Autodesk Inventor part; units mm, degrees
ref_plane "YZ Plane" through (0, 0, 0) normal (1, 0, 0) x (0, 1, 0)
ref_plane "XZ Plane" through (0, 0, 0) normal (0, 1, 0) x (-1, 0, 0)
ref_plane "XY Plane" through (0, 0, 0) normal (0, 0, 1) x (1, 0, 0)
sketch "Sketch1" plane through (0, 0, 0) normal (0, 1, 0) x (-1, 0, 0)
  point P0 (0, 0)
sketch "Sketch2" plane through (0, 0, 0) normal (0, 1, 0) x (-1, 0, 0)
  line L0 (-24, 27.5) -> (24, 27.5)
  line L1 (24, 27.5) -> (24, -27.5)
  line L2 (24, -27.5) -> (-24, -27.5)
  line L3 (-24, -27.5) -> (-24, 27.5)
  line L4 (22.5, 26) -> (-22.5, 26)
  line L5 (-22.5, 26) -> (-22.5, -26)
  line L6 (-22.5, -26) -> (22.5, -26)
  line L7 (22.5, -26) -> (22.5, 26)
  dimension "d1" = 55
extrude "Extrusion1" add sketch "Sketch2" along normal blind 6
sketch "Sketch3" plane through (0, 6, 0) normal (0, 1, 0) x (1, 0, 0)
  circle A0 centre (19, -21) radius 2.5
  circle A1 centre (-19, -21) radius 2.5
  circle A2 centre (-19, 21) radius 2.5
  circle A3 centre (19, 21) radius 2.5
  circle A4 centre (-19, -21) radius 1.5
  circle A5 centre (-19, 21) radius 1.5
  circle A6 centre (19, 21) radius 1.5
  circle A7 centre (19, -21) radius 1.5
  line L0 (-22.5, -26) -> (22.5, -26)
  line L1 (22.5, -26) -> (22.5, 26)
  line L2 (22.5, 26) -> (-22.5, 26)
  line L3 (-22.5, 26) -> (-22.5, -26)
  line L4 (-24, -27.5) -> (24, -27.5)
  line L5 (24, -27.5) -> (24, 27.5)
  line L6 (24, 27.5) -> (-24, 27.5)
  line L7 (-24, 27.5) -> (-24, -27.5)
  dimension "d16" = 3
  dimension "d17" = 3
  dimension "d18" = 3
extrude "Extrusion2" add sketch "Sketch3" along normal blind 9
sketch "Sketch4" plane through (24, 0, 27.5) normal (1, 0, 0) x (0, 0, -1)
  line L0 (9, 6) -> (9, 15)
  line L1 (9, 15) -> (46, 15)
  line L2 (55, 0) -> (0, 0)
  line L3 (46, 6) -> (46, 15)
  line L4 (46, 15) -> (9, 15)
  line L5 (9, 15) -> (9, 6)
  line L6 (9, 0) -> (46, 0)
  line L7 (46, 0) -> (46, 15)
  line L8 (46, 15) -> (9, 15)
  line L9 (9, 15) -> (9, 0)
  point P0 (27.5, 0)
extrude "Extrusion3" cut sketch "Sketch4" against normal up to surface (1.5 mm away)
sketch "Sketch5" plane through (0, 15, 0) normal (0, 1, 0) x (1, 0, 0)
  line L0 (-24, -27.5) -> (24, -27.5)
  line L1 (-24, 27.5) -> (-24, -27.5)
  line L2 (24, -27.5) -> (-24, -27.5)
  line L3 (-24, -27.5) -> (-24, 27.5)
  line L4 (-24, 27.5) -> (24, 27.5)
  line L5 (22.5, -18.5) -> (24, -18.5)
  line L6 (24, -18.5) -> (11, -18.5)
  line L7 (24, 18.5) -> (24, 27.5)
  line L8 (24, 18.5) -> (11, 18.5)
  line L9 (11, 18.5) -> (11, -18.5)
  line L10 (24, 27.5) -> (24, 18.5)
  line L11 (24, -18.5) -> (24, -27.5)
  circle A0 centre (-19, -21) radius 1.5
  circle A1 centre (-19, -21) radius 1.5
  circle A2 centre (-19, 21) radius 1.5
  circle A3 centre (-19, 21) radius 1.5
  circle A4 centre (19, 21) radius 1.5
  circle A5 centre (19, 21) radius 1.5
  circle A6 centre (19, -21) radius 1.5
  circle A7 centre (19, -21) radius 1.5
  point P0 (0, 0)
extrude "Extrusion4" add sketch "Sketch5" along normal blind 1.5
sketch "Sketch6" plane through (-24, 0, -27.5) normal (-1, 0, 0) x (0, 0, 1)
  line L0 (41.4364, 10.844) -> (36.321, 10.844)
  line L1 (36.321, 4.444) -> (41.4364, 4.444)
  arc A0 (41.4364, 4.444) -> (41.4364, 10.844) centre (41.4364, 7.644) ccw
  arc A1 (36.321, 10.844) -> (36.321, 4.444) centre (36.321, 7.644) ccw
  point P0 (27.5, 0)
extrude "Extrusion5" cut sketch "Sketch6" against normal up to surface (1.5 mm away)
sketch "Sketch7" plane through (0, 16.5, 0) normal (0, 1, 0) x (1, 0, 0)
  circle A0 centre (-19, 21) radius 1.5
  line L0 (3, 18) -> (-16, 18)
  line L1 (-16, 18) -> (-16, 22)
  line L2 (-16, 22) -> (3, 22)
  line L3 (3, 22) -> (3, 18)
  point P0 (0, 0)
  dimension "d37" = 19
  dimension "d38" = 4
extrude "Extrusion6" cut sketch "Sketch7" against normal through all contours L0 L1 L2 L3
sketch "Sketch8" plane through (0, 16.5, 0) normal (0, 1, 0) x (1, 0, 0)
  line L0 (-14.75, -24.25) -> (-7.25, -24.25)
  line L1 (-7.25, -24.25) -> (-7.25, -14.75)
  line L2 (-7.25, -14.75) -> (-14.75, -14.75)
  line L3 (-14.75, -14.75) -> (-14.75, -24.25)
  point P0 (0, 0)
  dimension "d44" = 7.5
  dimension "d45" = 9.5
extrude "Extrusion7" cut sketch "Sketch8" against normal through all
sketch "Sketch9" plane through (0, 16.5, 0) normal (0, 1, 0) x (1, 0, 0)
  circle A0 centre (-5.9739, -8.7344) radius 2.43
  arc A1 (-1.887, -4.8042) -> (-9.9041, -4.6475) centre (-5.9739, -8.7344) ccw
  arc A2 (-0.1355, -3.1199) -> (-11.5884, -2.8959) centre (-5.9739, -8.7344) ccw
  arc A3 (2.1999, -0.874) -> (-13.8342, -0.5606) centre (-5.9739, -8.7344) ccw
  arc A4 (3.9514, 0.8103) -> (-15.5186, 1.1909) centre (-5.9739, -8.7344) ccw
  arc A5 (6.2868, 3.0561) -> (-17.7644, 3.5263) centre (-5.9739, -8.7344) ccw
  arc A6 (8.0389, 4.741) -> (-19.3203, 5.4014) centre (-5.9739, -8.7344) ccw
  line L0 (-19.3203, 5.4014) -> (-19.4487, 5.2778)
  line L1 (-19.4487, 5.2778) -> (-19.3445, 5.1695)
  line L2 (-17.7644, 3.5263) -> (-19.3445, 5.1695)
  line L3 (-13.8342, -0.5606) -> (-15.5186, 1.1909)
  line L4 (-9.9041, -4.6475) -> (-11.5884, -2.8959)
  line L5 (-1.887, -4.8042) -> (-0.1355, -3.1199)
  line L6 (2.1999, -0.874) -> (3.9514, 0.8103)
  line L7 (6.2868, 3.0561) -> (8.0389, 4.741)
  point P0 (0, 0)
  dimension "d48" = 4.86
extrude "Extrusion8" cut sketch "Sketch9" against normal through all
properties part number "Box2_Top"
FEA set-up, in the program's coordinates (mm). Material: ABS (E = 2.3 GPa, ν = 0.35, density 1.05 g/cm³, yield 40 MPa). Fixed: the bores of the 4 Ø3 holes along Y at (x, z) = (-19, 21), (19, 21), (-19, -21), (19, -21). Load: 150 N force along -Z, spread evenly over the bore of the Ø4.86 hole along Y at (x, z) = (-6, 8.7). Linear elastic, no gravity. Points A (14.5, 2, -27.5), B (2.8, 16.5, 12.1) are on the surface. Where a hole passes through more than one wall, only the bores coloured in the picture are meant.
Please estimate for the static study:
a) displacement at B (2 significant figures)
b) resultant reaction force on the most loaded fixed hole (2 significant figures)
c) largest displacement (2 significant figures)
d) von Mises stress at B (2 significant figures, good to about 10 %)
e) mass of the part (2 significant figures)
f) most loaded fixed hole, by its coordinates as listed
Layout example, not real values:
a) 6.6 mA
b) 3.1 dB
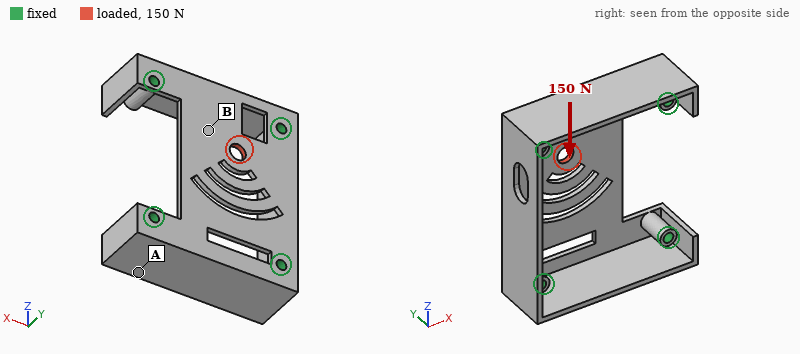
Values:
a) 0.088 mm
b) 79 N
c) 0.12 mm
d) 3.9 MPa
e) 7.1 g
f) (-19, 21)
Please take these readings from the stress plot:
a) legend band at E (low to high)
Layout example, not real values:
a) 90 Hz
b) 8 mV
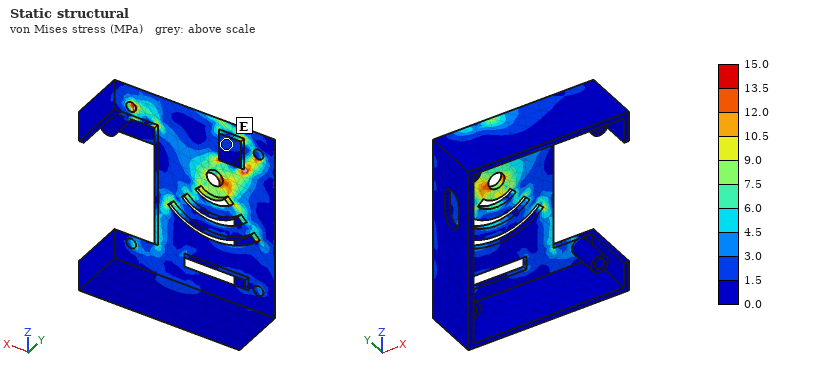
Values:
a) 1.5 to 3.0 MPa
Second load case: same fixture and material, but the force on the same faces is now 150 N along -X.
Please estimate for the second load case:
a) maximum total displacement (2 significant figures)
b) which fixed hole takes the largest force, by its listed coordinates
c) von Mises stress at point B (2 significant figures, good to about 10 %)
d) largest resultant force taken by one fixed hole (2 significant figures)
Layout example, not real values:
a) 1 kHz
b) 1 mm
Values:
a) 0.10 mm
b) (-19, 21)
c) 4.3 MPa
d) 75 N
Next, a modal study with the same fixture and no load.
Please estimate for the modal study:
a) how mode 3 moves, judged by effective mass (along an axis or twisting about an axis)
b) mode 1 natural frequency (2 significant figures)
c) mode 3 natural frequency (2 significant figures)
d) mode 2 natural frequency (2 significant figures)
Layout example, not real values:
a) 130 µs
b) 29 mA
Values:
a) along Z
b) 870 Hz
c) 1300 Hz
d) 1300 Hz
